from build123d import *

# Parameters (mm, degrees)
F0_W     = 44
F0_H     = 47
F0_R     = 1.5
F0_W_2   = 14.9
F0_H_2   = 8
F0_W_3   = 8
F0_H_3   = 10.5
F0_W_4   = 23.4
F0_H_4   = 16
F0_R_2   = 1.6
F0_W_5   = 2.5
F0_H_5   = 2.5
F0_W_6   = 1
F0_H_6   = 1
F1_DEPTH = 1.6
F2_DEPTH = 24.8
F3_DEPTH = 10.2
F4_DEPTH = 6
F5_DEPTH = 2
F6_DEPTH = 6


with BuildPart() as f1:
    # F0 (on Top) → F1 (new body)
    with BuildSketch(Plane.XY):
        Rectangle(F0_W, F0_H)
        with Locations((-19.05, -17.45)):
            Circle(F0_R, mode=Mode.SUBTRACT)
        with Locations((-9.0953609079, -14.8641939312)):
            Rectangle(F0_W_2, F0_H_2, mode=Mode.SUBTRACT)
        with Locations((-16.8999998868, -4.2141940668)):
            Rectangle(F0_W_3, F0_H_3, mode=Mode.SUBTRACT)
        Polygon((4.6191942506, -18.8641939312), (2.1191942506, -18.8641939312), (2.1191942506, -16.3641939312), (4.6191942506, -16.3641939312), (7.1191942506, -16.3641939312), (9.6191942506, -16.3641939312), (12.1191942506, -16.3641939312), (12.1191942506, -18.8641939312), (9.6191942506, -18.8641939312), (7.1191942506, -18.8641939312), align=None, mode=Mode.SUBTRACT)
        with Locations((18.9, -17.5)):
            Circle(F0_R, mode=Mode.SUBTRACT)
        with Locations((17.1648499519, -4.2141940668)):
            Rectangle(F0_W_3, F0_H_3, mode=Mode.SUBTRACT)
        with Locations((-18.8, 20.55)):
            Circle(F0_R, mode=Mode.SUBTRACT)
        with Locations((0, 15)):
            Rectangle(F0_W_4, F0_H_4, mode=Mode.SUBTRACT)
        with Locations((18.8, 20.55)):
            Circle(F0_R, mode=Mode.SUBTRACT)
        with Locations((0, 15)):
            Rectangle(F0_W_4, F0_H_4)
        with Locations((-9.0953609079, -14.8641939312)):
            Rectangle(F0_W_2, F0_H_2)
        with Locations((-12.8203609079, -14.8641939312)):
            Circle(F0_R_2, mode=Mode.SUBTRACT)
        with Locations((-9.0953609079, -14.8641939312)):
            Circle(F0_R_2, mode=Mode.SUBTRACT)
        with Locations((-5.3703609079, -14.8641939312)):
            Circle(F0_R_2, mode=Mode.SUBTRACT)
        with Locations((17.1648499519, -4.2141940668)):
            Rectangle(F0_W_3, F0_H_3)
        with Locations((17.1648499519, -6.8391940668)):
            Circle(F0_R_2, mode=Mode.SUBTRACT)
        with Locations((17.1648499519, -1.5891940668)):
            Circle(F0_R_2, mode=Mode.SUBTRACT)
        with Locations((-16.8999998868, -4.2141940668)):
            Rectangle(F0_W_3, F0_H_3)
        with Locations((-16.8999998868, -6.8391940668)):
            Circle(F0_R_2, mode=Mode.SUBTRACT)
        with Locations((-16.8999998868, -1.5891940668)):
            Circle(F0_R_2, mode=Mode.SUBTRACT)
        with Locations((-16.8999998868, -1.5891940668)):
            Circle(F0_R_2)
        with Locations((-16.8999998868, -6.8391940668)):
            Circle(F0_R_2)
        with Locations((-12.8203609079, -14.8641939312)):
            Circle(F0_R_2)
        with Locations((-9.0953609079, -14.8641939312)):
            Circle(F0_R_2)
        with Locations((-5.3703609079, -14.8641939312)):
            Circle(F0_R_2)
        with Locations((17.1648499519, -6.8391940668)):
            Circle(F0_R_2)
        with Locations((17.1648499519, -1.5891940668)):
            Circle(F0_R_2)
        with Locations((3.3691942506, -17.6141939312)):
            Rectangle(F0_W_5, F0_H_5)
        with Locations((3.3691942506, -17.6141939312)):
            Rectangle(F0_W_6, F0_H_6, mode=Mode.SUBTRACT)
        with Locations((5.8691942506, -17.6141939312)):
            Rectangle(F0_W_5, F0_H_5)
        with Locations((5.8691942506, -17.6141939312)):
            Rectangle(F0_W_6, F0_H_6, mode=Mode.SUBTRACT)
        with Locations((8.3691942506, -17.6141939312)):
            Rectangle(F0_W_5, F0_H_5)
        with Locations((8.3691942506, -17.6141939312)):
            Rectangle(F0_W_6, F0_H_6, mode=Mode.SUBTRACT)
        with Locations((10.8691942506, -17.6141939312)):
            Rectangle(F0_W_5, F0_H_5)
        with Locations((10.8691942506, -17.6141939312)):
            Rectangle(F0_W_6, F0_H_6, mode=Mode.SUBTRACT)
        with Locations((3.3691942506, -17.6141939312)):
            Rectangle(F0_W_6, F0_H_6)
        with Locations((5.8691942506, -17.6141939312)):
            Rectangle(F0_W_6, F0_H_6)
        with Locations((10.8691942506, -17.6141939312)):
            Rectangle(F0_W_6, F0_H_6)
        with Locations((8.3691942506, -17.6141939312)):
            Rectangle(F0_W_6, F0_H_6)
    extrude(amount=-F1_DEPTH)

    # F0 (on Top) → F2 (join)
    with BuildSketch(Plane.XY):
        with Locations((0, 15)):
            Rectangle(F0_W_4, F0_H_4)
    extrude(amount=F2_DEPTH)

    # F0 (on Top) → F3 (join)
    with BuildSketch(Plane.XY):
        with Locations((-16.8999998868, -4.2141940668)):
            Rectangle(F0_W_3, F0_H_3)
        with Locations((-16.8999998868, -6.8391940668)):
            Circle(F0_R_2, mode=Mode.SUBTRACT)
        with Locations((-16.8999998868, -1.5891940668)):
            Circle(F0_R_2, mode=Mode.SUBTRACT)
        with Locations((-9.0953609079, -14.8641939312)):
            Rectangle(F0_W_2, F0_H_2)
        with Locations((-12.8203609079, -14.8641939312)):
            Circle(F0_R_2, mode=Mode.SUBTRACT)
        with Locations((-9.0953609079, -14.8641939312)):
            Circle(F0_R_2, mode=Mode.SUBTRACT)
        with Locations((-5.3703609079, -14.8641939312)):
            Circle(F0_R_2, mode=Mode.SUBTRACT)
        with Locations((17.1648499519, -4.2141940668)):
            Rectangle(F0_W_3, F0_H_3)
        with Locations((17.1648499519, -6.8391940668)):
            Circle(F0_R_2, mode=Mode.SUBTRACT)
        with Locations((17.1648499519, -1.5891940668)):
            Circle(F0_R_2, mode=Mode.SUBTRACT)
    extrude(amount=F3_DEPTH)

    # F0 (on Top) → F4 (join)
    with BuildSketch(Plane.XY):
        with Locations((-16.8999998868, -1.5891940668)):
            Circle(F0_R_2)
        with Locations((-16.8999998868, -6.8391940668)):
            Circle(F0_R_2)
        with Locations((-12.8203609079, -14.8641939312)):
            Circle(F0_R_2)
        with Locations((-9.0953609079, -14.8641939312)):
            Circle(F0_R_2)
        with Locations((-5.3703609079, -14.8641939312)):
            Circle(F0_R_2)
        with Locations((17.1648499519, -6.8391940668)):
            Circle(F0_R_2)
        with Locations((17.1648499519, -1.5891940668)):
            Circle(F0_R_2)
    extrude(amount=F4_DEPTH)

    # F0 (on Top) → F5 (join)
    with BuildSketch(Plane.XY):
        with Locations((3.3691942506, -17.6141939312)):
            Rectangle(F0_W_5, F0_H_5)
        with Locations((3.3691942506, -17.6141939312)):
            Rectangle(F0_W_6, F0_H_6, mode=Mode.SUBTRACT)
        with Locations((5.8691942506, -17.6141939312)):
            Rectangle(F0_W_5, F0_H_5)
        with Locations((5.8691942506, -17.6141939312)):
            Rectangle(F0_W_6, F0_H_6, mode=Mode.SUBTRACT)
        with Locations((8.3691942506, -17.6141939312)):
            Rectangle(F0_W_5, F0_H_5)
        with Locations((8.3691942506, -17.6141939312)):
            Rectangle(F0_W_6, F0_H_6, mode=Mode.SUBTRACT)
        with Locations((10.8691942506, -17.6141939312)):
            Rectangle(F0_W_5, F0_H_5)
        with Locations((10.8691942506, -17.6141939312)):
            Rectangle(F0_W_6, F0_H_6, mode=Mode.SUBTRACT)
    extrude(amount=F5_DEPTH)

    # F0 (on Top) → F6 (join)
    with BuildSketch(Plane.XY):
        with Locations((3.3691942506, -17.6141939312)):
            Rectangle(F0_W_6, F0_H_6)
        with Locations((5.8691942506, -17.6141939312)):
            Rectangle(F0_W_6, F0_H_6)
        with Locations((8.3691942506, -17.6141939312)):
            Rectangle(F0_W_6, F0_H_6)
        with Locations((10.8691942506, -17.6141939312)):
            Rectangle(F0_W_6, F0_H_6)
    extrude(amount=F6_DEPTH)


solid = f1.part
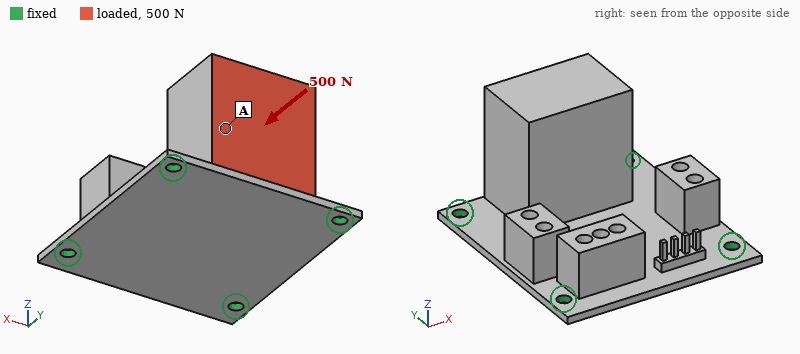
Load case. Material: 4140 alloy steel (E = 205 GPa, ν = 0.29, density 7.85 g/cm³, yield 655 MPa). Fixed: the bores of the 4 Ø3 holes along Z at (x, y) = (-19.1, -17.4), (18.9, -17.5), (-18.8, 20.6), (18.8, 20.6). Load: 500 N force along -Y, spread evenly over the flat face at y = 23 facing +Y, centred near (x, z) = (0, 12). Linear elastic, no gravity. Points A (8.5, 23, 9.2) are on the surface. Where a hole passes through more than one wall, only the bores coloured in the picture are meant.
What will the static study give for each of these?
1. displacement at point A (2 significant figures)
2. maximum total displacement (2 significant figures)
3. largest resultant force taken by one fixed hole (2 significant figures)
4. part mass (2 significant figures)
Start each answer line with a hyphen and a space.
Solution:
- 0.043 mm
- 0.11 mm
- 190 N
- 120 g
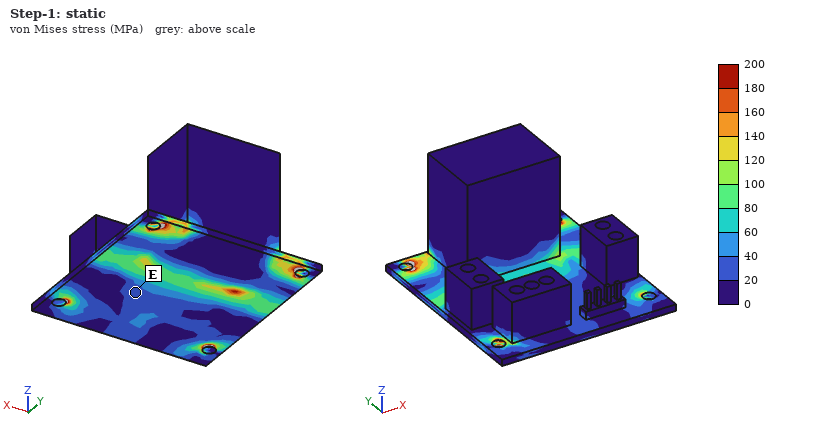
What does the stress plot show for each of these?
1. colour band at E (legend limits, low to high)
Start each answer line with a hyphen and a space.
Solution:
- 20 to 40 MPa
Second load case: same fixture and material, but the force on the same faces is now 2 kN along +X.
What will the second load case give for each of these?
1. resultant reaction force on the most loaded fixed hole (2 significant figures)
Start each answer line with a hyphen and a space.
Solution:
- 1.2 kN
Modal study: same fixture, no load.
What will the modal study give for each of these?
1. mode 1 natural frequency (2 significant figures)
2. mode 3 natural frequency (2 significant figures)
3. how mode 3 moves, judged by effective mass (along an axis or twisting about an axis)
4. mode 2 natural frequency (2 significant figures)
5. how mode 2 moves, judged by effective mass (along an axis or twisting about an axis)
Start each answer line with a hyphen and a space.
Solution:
- 1400 Hz
- 3600 Hz
- along Z
- 3300 Hz
- along X
